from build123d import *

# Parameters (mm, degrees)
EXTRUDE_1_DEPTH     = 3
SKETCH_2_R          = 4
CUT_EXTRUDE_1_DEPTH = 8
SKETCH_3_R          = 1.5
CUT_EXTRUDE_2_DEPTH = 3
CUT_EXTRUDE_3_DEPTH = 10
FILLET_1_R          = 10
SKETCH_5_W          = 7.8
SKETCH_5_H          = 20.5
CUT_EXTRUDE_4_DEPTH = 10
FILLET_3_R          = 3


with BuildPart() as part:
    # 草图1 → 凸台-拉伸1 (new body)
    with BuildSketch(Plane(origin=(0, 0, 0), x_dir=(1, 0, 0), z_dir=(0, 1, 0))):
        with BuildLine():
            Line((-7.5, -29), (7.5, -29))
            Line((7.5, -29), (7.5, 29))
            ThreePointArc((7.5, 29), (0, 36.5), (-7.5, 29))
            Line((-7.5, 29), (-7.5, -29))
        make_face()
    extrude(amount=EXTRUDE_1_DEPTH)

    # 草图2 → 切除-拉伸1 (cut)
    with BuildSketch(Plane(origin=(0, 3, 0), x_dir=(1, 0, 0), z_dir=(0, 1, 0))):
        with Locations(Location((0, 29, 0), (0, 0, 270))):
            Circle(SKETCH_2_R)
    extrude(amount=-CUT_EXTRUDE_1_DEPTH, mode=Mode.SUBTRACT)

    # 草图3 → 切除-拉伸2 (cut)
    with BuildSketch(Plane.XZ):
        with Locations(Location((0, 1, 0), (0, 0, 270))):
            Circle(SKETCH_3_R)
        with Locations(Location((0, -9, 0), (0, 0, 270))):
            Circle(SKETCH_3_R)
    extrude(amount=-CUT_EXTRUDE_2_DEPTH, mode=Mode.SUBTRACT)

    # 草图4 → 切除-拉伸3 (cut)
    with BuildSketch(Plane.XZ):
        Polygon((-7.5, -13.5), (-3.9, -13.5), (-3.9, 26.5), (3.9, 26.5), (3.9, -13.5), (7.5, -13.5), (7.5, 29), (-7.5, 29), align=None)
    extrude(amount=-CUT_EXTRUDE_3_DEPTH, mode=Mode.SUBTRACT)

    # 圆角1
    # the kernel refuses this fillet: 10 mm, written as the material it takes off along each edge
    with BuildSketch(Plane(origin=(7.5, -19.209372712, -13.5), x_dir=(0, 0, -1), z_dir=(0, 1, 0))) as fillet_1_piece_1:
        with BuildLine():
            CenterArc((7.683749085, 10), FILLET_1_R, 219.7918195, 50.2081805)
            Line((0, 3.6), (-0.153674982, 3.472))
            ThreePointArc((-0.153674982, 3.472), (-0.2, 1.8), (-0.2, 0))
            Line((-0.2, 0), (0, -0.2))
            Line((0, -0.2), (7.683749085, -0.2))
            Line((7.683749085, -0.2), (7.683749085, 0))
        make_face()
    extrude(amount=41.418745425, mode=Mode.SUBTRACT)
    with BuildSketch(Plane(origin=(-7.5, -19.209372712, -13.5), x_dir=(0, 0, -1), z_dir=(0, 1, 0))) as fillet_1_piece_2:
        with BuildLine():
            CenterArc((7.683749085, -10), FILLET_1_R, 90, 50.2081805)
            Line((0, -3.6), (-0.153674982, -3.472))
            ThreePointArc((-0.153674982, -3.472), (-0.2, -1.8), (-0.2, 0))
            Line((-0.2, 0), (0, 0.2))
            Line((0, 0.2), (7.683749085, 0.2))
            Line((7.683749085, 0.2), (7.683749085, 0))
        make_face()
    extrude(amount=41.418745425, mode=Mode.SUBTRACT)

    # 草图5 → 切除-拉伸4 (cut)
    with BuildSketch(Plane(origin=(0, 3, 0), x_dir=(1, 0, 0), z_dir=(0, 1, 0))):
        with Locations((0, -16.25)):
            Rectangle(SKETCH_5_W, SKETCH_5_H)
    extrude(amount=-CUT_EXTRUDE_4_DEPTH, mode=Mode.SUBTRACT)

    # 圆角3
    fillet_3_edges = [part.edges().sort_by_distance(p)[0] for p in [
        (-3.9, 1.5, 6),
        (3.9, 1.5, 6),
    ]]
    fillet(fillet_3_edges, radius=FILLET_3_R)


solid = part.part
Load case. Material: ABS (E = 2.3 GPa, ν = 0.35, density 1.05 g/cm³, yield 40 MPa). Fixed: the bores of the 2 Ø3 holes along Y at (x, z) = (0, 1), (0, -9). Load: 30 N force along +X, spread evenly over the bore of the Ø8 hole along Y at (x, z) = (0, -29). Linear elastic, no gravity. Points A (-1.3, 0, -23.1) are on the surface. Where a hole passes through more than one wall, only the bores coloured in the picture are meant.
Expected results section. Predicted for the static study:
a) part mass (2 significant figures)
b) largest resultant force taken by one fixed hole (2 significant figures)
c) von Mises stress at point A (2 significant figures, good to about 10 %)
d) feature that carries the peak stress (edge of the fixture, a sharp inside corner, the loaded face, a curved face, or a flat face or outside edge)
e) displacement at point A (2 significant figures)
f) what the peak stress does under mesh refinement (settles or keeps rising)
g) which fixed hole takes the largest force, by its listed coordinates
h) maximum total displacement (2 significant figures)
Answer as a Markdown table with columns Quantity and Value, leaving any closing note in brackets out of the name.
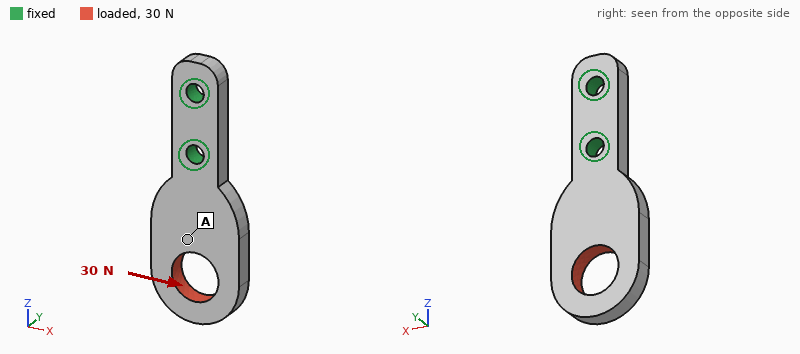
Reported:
| Quantity | Value |
|---|---|
| part mass | 1.2 g |
| largest resultant force taken by one fixed hole | 52 N |
| von Mises stress at point A | 3.0 MPa |
| feature that carries the peak stress | edge of the fixture |
| displacement at point A | 0.21 mm |
| what the peak stress does under mesh refinement | keeps rising |
| which fixed hole takes the largest force, by its listed coordinates | (0, -9) |
| maximum total displacement | 0.47 mm |
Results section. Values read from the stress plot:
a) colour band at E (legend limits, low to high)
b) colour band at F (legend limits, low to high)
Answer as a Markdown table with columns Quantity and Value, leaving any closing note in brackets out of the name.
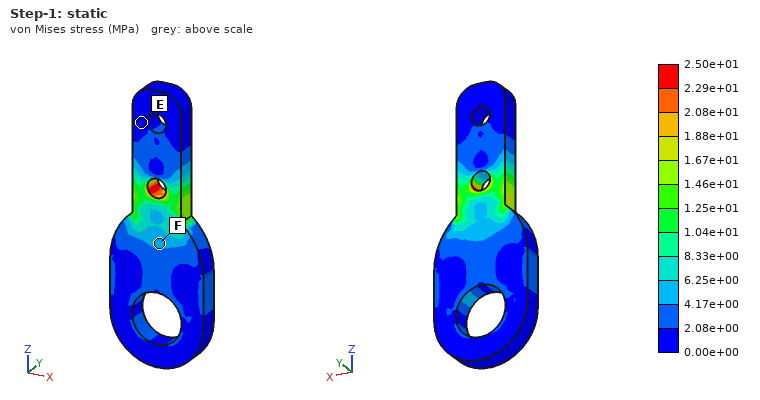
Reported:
| Quantity | Value |
|---|---|
| colour band at E | 0.00e+00 to 2.08e+00 MPa |
| colour band at F | 4.17e+00 to 6.25e+00 MPa |
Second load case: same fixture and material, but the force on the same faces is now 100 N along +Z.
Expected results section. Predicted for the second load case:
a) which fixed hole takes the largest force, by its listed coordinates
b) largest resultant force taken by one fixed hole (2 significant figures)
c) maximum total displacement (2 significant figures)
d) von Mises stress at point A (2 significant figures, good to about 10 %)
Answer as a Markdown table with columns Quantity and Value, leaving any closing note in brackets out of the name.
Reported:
| Quantity | Value |
|---|---|
| which fixed hole takes the largest force, by its listed coordinates | (0, -9) |
| largest resultant force taken by one fixed hole | 93 N |
| maximum total displacement | 48 µm |
| von Mises stress at point A | 2.4 MPa |
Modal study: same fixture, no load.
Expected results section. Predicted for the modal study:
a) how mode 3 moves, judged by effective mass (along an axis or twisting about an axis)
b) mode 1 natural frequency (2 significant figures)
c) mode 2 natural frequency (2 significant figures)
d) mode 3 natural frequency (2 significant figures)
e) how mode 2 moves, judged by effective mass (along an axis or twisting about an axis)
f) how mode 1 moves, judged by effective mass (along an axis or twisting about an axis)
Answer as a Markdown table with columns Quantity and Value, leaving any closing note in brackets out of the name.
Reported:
| Quantity | Value |
|---|---|
| how mode 3 moves, judged by effective mass | twisting about Z |
| mode 1 natural frequency | 1000 Hz |
| mode 2 natural frequency | 2100 Hz |
| mode 3 natural frequency | 2900 Hz |
| how mode 2 moves, judged by effective mass | along X |
| how mode 1 moves, judged by effective mass | along Y |
